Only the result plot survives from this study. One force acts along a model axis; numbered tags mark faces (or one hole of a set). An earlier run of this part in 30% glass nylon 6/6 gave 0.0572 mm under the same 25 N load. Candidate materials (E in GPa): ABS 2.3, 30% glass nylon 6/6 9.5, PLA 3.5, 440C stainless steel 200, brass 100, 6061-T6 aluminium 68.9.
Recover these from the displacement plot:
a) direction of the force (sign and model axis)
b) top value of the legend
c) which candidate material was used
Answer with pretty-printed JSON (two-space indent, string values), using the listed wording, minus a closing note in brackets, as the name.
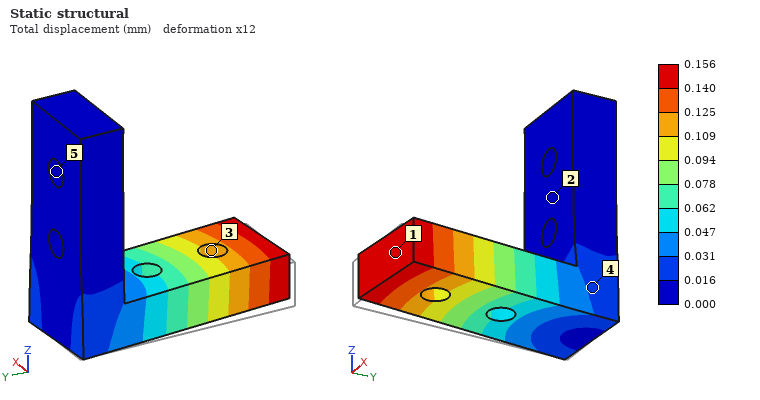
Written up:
{
  "direction of the force": "+X",
  "top value of the legend": "0.156 mm",
  "which candidate material was used": "PLA"
}
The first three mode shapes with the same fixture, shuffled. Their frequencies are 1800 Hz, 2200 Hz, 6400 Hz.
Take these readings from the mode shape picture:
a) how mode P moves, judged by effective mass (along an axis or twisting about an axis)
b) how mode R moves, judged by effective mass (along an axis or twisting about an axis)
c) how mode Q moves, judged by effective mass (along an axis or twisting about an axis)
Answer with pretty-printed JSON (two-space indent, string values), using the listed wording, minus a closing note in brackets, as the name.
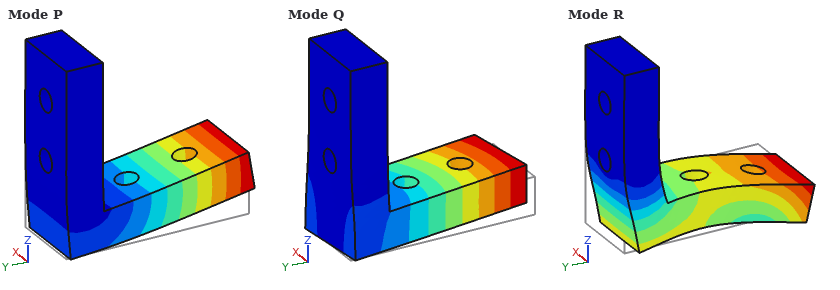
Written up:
{
  "how mode P moves, judged by effective mass": "along Z",
  "how mode R moves, judged by effective mass": "along Y",
  "how mode Q moves, judged by effective mass": "along X"
}
